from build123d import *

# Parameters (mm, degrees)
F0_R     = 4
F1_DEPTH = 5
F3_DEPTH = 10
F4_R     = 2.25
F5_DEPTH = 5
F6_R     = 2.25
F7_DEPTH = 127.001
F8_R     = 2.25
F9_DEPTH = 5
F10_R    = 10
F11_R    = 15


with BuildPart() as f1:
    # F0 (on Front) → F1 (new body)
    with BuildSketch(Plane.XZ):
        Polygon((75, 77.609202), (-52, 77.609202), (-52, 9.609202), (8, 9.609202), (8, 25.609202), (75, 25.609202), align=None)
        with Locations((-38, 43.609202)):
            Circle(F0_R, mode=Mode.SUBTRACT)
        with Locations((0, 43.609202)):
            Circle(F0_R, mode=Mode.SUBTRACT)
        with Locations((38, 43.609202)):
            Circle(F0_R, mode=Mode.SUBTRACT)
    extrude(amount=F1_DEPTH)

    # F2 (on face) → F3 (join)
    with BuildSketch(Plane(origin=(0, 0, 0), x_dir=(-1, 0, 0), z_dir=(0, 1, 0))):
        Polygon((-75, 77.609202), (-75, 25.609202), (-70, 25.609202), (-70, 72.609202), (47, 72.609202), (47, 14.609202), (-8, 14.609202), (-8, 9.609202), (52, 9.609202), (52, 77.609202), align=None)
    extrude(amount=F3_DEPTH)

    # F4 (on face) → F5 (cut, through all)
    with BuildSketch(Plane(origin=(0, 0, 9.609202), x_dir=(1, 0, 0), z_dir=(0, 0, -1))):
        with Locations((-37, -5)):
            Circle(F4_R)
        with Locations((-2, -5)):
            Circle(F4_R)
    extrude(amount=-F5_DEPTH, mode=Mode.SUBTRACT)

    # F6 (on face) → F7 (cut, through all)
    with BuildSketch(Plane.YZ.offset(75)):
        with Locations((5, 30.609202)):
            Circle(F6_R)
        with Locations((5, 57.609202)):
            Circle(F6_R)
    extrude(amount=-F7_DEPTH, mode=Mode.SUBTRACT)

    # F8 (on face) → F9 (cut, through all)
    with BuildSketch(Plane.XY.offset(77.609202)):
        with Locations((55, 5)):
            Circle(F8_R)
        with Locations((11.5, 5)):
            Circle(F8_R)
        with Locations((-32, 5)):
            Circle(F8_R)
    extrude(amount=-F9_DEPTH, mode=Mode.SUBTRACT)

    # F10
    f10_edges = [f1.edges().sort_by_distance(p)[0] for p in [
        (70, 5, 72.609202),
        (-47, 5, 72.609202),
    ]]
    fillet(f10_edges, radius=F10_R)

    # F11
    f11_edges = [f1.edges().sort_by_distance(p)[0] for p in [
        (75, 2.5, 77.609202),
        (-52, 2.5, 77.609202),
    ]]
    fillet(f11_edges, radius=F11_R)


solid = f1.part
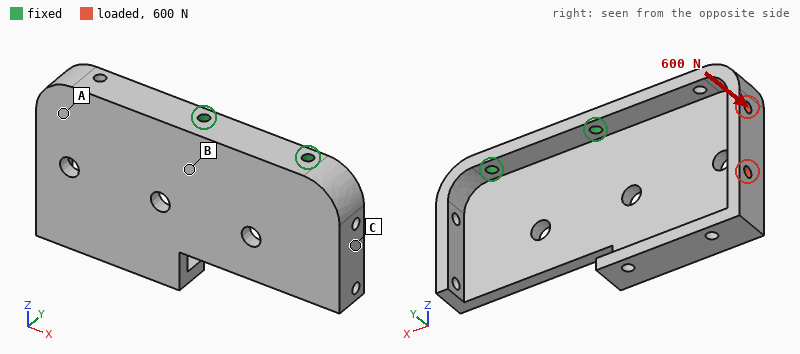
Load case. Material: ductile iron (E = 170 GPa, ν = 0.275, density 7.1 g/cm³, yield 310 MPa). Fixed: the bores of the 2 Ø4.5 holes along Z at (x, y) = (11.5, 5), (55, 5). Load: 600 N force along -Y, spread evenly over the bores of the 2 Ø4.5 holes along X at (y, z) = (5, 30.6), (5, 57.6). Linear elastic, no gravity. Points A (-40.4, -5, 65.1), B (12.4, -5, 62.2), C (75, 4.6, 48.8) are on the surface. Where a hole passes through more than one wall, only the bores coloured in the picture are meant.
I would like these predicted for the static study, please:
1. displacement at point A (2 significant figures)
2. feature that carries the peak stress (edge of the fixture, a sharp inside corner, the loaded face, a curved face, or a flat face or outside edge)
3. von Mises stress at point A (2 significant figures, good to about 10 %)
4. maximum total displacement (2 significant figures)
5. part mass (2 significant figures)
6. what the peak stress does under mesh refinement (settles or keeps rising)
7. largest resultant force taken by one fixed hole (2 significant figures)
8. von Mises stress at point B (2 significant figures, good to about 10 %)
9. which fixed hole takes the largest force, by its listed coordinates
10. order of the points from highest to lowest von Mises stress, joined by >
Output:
0.18 mm
edge of the fixture
29 MPa
0.61 mm
350 g
keeps rising
1.6 kN
67 MPa
(11.5, 5)
B > A > C
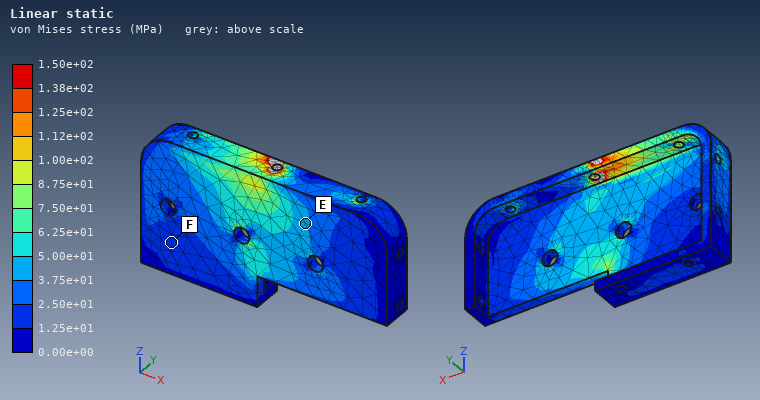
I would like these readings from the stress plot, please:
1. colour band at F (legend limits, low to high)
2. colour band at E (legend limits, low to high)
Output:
1.25e+01 to 2.50e+01 MPa
3.75e+01 to 5.00e+01 MPa
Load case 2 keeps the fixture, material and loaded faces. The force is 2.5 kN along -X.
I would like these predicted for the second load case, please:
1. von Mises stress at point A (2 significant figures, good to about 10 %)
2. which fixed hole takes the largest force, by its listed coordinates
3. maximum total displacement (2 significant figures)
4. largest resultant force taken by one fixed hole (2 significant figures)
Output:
27 MPa
(11.5, 5)
0.24 mm
2.5 kN
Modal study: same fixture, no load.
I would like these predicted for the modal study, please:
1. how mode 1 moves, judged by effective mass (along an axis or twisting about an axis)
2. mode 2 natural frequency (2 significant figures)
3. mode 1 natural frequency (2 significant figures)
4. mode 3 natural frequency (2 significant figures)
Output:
along Y
1300 Hz
510 Hz
2000 Hz
